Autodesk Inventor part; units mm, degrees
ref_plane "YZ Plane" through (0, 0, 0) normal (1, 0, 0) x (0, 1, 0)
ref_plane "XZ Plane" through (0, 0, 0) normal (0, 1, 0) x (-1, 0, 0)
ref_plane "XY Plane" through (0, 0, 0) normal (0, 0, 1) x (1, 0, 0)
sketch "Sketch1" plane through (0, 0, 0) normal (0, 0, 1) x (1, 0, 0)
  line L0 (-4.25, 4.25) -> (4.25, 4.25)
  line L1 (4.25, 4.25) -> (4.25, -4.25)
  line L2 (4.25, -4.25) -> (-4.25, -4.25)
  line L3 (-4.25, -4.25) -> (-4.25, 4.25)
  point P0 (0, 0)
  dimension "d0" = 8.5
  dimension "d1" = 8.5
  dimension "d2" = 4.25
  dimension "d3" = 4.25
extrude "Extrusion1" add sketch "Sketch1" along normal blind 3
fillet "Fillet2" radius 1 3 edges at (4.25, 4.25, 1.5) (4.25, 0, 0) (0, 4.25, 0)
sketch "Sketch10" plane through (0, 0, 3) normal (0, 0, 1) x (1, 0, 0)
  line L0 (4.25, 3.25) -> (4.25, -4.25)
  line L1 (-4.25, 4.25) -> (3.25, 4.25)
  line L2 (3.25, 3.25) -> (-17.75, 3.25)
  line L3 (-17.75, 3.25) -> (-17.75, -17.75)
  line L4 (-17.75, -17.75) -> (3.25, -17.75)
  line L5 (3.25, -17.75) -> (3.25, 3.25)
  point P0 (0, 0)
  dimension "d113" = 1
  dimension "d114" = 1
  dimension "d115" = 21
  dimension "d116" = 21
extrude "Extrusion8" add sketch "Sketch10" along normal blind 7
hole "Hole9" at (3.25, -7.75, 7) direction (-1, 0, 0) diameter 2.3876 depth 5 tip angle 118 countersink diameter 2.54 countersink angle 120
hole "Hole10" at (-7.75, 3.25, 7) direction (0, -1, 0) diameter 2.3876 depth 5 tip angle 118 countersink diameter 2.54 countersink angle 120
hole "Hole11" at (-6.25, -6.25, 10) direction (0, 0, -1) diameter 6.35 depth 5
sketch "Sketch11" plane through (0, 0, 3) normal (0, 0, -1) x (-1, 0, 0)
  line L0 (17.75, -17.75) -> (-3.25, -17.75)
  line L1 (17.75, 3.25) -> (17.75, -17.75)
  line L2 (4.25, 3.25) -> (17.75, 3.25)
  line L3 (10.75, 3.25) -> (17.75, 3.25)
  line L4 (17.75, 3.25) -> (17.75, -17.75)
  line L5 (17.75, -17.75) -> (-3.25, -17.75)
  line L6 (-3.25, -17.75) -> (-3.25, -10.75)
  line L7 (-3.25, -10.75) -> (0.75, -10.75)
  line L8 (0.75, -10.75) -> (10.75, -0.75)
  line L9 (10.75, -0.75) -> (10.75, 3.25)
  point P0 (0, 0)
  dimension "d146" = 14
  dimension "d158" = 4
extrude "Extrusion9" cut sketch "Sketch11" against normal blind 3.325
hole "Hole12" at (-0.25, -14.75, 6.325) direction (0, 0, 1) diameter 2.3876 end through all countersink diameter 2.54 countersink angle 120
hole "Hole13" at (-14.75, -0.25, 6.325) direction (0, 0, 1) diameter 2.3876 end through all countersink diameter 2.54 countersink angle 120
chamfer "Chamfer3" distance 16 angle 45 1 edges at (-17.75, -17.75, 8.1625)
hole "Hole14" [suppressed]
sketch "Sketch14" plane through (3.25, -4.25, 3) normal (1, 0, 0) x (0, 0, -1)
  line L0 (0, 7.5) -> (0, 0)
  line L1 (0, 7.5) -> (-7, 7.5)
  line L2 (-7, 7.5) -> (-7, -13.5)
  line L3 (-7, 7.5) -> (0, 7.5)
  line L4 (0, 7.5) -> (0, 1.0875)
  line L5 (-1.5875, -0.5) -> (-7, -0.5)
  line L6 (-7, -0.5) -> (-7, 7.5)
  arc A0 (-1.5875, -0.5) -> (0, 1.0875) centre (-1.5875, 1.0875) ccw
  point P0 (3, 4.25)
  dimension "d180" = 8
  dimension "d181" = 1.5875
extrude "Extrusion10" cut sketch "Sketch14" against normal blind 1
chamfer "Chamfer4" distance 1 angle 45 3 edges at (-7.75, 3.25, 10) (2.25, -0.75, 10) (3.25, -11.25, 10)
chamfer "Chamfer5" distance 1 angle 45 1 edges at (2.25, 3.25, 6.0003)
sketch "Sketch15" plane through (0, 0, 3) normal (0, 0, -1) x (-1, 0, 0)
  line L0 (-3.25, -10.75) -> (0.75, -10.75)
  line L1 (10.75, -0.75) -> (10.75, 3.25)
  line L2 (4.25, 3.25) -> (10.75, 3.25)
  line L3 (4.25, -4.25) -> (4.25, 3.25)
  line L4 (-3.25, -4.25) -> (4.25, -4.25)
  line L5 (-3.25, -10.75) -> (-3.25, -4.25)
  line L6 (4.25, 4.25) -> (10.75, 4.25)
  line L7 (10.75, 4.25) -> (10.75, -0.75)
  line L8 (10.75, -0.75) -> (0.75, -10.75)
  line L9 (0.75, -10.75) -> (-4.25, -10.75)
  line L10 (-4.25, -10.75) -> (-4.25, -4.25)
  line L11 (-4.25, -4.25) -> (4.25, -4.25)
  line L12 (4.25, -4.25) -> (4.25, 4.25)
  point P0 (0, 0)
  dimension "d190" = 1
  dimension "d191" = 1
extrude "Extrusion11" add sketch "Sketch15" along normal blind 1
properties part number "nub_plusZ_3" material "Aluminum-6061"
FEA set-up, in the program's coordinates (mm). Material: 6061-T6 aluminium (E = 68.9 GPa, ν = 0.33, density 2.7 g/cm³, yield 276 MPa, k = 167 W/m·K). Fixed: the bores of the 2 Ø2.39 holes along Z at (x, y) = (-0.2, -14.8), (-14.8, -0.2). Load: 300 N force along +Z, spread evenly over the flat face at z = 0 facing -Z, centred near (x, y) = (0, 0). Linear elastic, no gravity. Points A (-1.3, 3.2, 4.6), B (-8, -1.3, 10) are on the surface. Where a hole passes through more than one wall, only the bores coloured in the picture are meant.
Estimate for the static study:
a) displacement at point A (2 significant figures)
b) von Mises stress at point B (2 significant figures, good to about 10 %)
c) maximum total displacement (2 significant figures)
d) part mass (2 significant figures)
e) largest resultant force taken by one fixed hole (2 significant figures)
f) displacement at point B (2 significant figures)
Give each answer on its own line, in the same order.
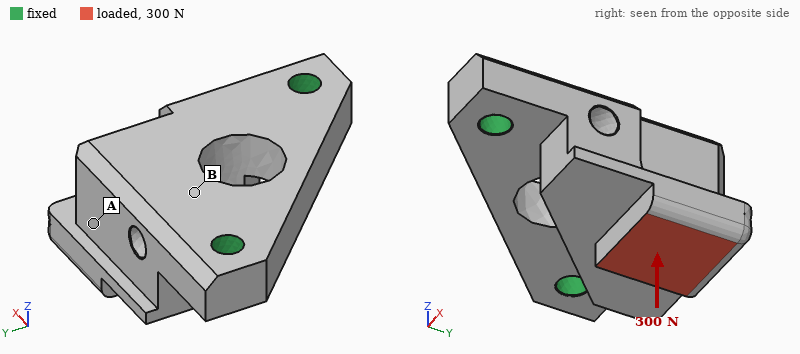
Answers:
38 µm
40 MPa
56 µm
4.5 g
160 N
9.9 µm
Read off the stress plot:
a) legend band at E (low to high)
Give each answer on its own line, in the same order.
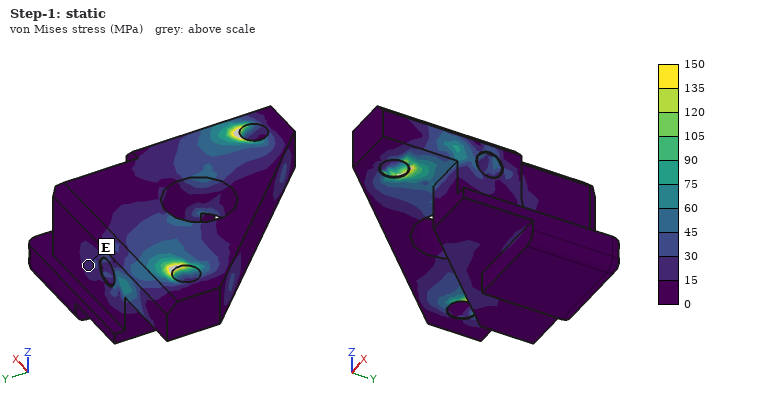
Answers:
15 to 30 MPa
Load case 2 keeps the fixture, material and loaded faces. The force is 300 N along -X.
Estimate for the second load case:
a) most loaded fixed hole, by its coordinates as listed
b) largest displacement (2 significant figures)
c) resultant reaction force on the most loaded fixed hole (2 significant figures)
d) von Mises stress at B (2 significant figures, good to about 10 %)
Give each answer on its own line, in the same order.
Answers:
(-14.8, -0.2)
42 µm
260 N
32 MPa
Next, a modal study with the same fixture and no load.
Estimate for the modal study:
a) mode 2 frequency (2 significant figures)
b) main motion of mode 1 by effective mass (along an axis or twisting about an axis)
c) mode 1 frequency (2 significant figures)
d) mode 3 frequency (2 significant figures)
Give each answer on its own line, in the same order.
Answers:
35 kHz
along Z
9900 Hz
36 kHz
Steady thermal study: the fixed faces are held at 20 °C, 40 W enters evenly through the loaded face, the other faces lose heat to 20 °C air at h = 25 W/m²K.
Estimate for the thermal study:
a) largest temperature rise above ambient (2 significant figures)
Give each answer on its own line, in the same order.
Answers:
62 K
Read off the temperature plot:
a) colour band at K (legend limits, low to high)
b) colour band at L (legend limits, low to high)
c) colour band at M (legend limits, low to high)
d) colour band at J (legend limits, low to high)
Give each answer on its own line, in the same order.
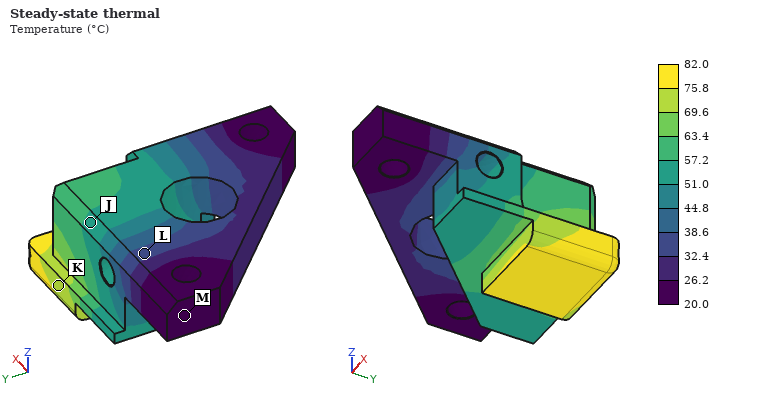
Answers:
69.6 to 75.8 °C
32.4 to 38.6 °C
20.0 to 26.2 °C
51.0 to 57.2 °C
